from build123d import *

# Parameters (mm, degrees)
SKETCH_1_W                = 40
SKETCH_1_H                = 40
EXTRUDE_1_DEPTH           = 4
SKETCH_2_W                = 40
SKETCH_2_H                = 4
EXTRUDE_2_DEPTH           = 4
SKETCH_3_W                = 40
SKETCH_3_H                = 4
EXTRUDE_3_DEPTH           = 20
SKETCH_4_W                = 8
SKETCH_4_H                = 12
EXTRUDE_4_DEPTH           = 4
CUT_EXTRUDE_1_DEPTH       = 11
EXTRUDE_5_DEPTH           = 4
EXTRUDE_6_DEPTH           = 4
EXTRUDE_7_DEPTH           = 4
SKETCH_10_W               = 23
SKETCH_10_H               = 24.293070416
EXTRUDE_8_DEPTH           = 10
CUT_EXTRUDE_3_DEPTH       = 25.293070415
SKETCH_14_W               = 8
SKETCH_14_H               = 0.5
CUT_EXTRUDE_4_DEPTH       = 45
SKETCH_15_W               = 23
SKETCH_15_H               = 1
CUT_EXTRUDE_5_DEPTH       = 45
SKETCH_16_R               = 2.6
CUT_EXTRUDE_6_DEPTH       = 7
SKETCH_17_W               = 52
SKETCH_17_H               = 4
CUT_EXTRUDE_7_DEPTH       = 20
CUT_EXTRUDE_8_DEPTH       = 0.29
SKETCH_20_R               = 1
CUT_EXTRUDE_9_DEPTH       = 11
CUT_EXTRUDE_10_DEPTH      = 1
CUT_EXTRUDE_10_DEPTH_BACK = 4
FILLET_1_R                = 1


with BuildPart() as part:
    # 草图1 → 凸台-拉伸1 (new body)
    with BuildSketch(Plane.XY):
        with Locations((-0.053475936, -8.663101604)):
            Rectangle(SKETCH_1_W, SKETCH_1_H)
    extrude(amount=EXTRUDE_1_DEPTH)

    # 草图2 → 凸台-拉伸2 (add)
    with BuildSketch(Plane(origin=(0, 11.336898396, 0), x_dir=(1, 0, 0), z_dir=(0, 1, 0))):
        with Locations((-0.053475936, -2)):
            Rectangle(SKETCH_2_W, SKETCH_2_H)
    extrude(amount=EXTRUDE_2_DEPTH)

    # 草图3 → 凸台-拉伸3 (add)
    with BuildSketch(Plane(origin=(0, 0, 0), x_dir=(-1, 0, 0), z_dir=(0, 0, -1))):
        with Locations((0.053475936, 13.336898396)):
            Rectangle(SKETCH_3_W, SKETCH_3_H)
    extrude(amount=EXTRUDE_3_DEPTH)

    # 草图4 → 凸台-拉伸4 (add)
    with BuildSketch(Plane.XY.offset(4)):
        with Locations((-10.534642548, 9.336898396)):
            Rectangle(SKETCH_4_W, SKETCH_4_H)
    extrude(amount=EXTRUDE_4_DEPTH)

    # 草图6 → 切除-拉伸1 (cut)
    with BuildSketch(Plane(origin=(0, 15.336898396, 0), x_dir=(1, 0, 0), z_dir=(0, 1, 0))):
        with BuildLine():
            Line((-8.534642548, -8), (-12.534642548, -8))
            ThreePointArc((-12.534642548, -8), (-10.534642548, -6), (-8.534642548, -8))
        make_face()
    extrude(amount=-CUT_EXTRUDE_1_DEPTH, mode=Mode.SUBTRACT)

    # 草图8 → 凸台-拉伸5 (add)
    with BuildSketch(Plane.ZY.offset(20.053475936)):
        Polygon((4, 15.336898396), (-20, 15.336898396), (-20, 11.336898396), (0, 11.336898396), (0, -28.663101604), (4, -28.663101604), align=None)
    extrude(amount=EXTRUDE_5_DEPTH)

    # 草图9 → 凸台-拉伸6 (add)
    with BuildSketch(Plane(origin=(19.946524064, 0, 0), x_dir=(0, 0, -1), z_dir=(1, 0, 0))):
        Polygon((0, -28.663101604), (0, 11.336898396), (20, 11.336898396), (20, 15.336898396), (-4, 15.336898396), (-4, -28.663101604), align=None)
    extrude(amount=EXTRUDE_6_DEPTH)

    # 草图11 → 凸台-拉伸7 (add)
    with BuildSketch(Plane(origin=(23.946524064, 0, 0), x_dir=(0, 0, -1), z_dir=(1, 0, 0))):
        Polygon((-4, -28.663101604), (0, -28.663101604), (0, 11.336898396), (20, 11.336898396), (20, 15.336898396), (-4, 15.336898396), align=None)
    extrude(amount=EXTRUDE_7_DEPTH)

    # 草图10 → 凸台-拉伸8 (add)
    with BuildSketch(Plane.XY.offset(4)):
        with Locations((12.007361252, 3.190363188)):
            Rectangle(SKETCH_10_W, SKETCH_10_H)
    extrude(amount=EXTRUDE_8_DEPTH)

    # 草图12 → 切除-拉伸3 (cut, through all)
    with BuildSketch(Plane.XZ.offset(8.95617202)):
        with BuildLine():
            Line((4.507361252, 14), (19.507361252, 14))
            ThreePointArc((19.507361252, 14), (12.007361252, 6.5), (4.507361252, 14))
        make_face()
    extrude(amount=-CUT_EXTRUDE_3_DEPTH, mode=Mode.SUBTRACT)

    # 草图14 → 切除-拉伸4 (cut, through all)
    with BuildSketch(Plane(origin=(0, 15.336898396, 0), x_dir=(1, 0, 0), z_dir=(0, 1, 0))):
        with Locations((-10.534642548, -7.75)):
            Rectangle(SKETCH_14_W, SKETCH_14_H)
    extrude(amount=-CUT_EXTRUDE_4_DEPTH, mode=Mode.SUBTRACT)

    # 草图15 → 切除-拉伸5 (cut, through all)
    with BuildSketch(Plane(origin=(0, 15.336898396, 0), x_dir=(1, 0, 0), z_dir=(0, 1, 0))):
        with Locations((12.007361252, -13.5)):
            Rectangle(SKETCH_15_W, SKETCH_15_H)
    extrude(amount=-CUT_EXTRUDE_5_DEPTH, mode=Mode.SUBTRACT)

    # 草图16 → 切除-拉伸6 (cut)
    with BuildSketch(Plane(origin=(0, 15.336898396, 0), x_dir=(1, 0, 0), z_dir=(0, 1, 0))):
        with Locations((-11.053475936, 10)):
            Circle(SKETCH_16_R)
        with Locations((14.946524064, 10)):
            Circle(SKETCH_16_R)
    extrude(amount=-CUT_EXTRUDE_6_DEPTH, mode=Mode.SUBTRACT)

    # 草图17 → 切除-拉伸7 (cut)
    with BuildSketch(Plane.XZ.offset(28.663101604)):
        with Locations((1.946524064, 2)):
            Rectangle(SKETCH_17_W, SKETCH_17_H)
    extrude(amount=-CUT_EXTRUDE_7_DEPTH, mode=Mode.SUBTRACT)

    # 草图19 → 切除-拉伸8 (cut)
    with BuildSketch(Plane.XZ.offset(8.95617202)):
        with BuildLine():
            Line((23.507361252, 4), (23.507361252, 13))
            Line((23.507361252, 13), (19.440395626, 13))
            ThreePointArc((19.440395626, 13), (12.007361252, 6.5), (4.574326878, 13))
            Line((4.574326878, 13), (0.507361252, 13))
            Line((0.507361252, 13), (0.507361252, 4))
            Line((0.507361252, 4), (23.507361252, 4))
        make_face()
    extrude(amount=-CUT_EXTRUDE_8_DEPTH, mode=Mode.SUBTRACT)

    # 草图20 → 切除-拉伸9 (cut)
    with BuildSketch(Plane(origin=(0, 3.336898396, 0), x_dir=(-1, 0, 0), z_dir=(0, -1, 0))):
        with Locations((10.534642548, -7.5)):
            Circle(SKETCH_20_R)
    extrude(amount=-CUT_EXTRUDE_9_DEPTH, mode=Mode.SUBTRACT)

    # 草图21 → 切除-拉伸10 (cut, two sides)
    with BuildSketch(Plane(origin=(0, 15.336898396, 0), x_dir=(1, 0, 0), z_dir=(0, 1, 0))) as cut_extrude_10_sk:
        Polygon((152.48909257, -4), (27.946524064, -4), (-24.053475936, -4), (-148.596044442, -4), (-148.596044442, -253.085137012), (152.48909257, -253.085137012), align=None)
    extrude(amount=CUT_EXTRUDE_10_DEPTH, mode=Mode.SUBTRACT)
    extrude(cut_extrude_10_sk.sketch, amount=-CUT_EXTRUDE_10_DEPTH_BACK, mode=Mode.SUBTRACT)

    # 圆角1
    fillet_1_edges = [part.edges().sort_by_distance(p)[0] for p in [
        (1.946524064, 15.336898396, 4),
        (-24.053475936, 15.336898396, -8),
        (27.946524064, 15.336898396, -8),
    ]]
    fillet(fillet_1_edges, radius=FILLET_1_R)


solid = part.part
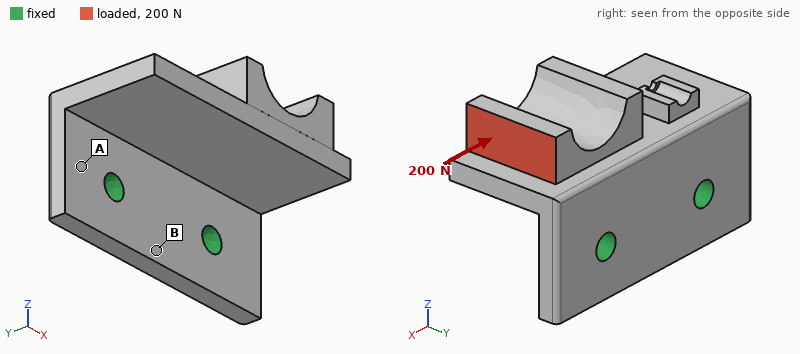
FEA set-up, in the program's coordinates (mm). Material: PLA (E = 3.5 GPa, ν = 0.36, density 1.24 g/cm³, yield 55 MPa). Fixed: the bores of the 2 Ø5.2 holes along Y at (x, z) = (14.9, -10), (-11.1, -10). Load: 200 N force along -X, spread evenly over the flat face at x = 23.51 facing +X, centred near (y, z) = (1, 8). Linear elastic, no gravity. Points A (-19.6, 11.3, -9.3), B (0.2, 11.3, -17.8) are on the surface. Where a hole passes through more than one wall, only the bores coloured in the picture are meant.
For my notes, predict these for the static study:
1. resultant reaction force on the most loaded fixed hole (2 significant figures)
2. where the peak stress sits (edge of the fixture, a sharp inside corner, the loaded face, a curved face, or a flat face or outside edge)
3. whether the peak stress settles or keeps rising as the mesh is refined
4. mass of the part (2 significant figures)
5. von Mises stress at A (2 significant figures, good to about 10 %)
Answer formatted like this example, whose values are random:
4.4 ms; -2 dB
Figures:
180 N; edge of the fixture; keeps rising; 15 g; 2.8 MPa
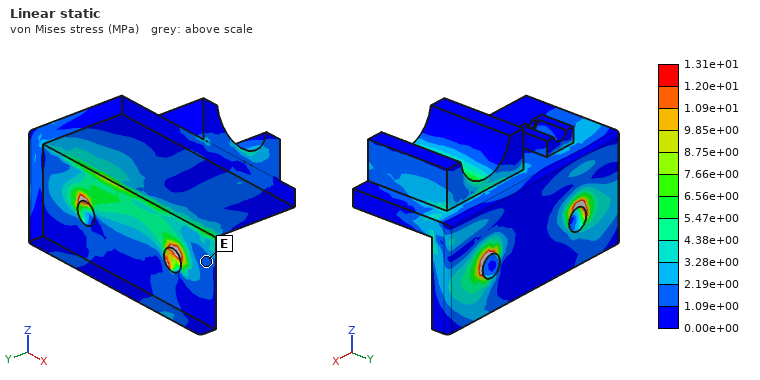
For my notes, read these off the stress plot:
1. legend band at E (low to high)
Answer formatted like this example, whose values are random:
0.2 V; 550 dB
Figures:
1.09e+00 to 2.19e+00 MPa
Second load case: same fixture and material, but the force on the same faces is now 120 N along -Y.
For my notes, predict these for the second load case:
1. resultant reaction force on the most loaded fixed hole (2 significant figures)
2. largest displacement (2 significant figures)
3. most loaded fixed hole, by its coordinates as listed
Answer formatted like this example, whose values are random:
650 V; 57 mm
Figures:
140 N; 0.75 mm; (14.9, -10)
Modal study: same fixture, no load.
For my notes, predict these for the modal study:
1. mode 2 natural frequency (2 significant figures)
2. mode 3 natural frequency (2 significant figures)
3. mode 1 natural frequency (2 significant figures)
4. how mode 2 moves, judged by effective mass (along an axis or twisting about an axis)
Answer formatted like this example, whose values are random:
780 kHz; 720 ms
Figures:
2000 Hz; 3100 Hz; 920 Hz; along X
